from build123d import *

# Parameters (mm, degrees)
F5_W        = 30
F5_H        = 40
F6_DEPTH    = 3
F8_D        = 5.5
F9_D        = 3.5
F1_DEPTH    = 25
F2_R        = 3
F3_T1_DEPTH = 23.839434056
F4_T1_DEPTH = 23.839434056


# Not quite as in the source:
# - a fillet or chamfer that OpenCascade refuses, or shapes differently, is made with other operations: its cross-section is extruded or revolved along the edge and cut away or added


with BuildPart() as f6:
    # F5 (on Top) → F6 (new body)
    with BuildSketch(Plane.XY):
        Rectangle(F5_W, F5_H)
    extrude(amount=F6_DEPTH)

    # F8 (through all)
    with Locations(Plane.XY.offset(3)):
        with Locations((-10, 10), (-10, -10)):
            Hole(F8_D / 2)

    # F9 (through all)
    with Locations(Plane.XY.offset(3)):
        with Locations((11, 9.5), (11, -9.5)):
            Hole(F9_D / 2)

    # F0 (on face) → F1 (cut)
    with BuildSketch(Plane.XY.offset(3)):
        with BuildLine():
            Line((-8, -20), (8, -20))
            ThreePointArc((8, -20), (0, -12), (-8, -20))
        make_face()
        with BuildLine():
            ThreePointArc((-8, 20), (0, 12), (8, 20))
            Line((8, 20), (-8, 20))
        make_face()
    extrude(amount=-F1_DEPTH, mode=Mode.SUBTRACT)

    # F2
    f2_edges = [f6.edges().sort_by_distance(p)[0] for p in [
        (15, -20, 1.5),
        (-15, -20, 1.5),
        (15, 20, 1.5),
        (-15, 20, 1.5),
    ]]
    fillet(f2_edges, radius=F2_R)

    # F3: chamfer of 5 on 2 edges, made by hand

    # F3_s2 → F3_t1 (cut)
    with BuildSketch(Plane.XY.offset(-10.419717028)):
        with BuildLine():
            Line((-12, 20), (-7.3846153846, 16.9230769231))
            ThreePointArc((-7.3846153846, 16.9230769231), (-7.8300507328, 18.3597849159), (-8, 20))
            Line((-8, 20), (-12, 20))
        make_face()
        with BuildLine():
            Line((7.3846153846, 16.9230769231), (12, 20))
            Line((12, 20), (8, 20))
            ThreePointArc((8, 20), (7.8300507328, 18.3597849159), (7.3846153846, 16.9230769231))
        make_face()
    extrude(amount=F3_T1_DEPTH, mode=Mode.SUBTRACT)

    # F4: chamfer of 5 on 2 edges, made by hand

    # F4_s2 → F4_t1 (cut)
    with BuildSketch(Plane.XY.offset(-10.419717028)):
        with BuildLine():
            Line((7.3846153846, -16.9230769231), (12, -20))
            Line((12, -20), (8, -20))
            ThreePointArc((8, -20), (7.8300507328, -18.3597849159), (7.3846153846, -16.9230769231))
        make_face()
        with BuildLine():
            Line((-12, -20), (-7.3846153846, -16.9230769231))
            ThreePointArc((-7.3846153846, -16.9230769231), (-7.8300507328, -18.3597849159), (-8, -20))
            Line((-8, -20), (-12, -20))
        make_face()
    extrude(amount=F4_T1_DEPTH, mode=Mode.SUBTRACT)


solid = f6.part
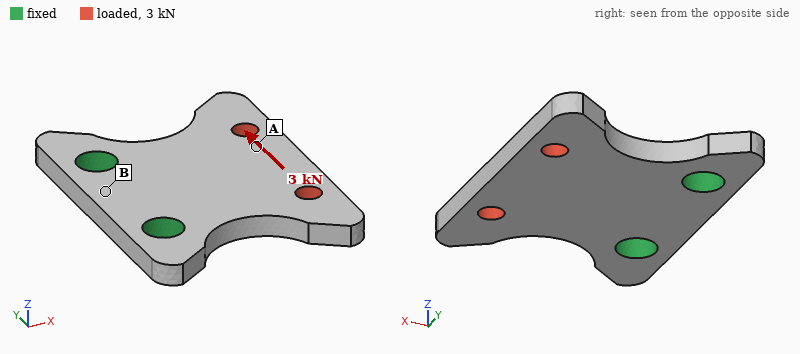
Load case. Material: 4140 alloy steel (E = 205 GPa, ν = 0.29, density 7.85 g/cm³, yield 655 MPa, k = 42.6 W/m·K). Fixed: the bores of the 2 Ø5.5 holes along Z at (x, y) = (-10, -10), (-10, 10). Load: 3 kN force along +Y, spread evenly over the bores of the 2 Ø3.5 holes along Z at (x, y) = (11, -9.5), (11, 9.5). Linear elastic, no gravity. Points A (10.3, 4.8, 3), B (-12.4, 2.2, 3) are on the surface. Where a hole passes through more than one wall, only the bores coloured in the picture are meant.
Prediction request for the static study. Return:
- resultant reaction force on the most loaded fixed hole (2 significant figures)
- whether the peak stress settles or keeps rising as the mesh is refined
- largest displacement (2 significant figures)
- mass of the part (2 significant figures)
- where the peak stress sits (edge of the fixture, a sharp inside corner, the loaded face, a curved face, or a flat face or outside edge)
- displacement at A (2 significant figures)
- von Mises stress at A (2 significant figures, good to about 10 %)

3.1 kN
keeps rising
28 µm
21 g
edge of the fixture
17 µm
65 MPa
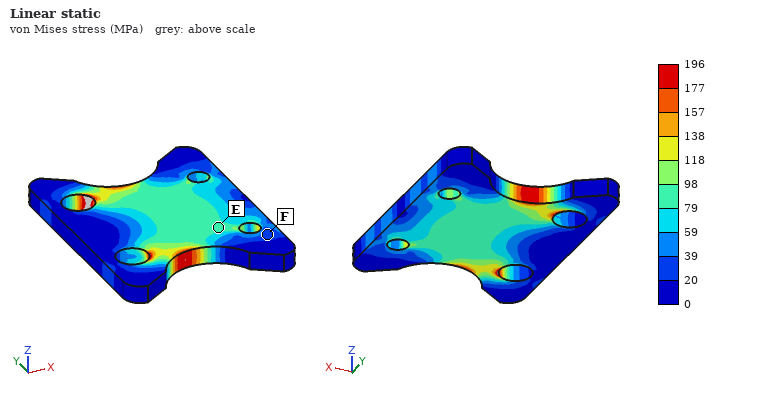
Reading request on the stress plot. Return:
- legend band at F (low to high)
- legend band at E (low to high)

20 to 39 MPa
79 to 98 MPa
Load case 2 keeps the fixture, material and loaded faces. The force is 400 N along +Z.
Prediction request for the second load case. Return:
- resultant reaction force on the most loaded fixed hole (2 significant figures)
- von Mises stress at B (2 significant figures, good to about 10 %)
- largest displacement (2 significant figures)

200 N
25 MPa
0.11 mm
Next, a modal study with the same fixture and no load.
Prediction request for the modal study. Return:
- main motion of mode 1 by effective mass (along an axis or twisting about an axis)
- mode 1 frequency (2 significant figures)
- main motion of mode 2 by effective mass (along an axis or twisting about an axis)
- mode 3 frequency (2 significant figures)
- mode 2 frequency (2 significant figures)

along Z
3900 Hz
twisting about X
14 kHz
6400 Hz
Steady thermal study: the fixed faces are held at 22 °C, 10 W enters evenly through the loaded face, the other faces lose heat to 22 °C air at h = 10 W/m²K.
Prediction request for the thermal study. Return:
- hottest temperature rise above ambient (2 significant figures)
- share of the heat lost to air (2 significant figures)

67 K
6.5 %
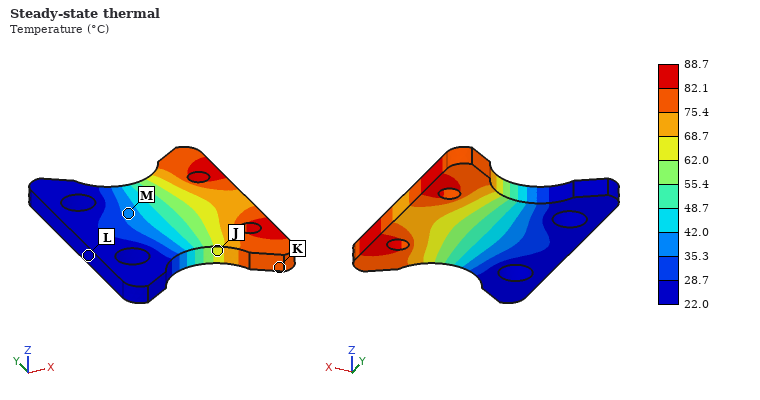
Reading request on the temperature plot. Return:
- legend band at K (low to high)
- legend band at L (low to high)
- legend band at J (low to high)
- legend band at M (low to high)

75.4 to 82.1 °C
22.0 to 28.7 °C
62.0 to 68.7 °C
35.3 to 42.0 °C
